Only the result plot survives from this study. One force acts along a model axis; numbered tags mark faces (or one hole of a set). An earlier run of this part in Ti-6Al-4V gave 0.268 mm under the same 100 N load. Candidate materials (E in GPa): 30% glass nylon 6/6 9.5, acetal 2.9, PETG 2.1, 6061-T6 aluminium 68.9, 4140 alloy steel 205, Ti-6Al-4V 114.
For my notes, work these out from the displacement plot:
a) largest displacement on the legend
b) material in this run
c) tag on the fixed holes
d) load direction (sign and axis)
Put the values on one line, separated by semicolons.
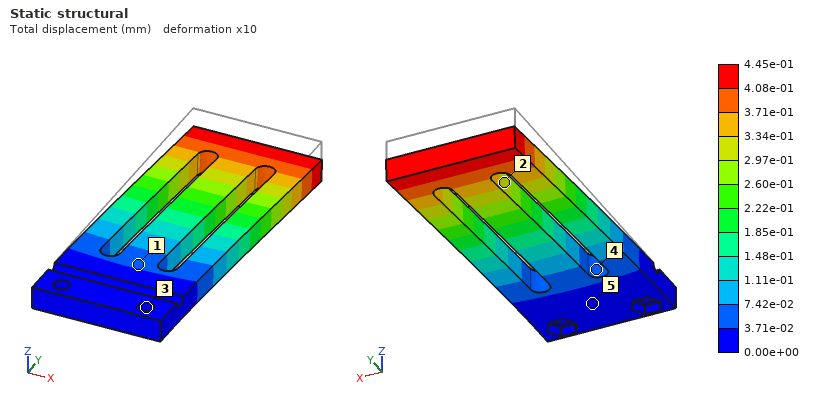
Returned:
4.45e-01 mm; 6061-T6 aluminium; 3; -Z
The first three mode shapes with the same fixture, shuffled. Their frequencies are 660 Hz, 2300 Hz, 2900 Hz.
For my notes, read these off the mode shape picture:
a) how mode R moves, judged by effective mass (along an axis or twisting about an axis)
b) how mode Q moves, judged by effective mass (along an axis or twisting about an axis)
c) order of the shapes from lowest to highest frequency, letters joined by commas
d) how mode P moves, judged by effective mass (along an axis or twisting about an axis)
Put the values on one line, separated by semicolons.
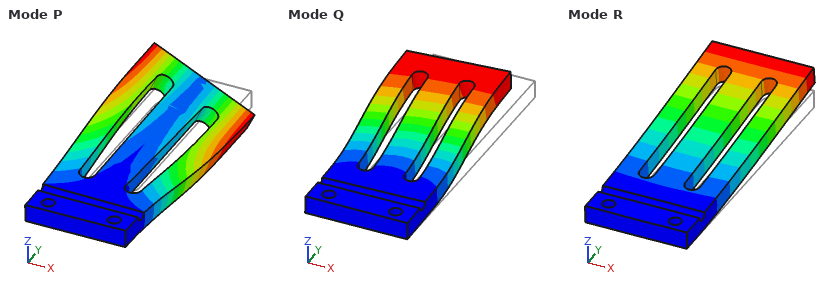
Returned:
along Z; along X; R, Q, P; twisting about Y
